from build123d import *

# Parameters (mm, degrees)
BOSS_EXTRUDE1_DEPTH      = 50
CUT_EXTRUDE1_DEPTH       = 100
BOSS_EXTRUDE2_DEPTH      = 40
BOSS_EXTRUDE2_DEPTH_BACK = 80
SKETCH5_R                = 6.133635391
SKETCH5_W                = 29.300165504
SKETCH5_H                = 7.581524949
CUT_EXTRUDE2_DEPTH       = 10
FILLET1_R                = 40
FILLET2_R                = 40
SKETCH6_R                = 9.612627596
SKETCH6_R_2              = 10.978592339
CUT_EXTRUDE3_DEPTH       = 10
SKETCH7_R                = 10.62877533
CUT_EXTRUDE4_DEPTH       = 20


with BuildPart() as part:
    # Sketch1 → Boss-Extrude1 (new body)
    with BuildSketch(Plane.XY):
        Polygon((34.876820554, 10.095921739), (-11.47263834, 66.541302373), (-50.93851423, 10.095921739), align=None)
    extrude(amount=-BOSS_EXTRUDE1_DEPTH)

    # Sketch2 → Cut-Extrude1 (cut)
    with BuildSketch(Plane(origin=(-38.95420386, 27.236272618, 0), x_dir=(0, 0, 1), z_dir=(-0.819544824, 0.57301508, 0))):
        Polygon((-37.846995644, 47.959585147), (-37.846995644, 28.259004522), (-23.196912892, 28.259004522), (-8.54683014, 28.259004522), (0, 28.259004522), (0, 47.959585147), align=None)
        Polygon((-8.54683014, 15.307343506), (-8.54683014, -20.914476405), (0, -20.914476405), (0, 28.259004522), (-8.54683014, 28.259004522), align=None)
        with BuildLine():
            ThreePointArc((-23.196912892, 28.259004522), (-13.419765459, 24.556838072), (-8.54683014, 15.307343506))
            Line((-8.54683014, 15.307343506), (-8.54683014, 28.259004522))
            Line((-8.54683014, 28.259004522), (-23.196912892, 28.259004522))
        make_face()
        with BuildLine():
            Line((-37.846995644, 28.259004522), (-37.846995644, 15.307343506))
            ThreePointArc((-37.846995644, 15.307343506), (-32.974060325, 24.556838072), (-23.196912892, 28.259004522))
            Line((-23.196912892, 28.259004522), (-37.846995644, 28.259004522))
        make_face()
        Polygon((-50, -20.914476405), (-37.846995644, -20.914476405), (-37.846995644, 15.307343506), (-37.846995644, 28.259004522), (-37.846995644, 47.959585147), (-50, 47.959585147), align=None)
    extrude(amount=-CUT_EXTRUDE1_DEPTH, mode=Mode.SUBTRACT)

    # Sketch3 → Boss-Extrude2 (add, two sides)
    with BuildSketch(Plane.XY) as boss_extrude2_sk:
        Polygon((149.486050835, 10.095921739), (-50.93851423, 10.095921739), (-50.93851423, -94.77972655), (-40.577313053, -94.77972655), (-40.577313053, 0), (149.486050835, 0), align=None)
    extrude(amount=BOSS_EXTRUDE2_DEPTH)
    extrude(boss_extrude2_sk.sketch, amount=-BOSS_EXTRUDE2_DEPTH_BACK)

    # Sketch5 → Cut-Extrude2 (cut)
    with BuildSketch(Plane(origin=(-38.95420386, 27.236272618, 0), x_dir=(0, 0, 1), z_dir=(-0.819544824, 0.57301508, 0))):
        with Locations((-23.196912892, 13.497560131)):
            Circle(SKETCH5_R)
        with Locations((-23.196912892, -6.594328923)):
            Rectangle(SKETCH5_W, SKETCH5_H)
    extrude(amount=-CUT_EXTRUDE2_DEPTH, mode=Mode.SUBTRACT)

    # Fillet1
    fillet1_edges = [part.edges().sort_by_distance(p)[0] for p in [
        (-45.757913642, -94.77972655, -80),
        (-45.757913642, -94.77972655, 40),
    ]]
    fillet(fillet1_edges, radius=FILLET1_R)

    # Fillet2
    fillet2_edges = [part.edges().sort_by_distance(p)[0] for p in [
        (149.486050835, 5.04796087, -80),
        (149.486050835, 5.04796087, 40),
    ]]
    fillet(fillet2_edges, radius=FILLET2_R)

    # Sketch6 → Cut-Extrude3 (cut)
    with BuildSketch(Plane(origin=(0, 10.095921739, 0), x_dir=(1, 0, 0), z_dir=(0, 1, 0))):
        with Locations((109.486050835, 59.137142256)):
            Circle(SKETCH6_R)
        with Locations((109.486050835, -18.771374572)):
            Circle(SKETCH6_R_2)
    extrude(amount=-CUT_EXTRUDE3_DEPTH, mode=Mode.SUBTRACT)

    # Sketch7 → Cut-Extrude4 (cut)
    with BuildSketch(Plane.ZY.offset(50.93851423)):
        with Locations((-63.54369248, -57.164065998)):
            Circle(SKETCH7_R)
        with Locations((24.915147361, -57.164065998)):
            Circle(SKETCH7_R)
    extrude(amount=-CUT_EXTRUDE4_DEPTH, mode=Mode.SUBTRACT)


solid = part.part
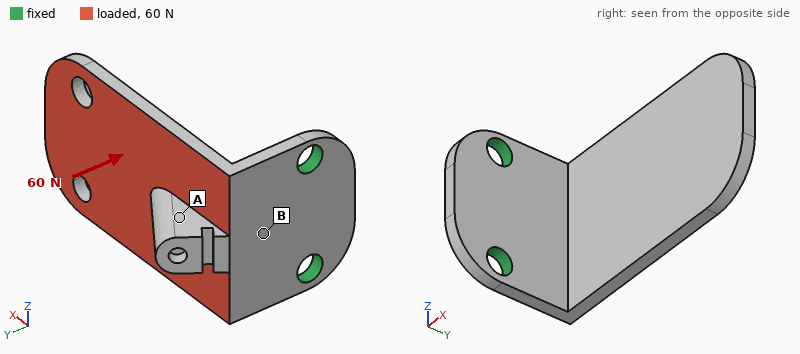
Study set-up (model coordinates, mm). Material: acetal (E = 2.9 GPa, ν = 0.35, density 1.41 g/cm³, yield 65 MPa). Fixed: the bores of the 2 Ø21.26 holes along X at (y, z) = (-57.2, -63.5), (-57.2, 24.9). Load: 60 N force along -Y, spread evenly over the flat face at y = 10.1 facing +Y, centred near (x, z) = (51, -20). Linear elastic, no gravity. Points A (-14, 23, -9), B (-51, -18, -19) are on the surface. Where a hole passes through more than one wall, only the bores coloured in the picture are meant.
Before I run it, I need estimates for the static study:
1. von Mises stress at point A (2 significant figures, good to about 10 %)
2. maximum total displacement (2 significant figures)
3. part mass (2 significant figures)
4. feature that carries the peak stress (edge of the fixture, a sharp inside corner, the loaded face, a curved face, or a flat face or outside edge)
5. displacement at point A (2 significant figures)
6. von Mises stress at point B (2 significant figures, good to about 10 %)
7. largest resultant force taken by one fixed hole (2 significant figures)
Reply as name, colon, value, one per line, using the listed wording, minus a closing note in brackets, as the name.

von Mises stress at point A: 0.44 MPa
maximum total displacement: 2.7 mm
part mass: 530 g
feature that carries the peak stress: a flat face or outside edge
displacement at point A: 0.60 mm
von Mises stress at point B: 2.4 MPa
largest resultant force taken by one fixed hole: 32 N
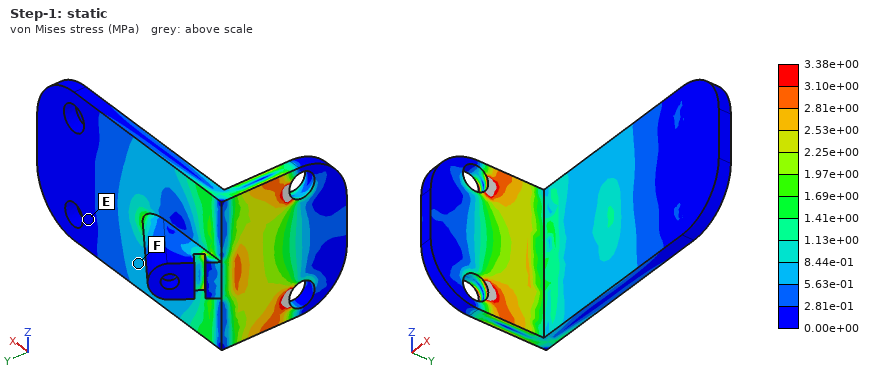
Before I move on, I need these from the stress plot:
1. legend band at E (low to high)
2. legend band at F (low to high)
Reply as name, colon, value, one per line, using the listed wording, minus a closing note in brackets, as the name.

legend band at E: 0.00e+00 to 2.81e-01 MPa
legend band at F: 5.63e-01 to 8.44e-01 MPa
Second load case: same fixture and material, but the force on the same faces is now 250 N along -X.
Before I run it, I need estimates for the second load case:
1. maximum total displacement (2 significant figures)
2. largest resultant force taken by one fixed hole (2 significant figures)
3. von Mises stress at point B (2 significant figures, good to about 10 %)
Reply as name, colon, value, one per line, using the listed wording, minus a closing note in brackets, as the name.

maximum total displacement: 3.0 mm
largest resultant force taken by one fixed hole: 130 N
von Mises stress at point B: 2.8 MPa
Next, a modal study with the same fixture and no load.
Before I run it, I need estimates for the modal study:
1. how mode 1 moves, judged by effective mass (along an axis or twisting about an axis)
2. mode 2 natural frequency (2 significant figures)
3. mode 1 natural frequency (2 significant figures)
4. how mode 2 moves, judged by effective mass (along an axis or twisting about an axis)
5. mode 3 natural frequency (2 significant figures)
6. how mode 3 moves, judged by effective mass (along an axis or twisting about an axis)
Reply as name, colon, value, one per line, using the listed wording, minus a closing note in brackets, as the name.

how mode 1 moves, judged by effective mass: along Y
mode 2 natural frequency: 120 Hz
mode 1 natural frequency: 53 Hz
how mode 2 moves, judged by effective mass: along Z
mode 3 natural frequency: 240 Hz
how mode 3 moves, judged by effective mass: along X
